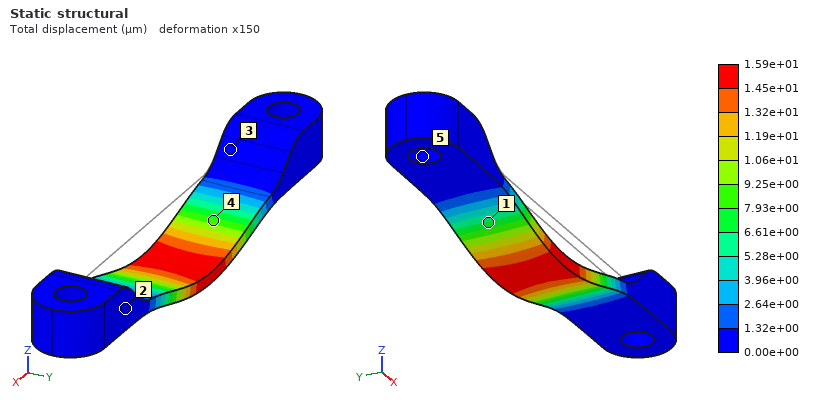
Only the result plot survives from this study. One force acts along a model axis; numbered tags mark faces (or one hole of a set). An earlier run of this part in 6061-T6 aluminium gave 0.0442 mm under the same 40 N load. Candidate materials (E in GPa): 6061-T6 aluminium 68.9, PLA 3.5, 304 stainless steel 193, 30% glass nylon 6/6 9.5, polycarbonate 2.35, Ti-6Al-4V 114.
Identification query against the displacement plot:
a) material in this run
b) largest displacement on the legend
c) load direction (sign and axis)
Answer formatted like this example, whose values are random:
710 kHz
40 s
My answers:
304 stainless steel
1.59e+01 µm
-Z
